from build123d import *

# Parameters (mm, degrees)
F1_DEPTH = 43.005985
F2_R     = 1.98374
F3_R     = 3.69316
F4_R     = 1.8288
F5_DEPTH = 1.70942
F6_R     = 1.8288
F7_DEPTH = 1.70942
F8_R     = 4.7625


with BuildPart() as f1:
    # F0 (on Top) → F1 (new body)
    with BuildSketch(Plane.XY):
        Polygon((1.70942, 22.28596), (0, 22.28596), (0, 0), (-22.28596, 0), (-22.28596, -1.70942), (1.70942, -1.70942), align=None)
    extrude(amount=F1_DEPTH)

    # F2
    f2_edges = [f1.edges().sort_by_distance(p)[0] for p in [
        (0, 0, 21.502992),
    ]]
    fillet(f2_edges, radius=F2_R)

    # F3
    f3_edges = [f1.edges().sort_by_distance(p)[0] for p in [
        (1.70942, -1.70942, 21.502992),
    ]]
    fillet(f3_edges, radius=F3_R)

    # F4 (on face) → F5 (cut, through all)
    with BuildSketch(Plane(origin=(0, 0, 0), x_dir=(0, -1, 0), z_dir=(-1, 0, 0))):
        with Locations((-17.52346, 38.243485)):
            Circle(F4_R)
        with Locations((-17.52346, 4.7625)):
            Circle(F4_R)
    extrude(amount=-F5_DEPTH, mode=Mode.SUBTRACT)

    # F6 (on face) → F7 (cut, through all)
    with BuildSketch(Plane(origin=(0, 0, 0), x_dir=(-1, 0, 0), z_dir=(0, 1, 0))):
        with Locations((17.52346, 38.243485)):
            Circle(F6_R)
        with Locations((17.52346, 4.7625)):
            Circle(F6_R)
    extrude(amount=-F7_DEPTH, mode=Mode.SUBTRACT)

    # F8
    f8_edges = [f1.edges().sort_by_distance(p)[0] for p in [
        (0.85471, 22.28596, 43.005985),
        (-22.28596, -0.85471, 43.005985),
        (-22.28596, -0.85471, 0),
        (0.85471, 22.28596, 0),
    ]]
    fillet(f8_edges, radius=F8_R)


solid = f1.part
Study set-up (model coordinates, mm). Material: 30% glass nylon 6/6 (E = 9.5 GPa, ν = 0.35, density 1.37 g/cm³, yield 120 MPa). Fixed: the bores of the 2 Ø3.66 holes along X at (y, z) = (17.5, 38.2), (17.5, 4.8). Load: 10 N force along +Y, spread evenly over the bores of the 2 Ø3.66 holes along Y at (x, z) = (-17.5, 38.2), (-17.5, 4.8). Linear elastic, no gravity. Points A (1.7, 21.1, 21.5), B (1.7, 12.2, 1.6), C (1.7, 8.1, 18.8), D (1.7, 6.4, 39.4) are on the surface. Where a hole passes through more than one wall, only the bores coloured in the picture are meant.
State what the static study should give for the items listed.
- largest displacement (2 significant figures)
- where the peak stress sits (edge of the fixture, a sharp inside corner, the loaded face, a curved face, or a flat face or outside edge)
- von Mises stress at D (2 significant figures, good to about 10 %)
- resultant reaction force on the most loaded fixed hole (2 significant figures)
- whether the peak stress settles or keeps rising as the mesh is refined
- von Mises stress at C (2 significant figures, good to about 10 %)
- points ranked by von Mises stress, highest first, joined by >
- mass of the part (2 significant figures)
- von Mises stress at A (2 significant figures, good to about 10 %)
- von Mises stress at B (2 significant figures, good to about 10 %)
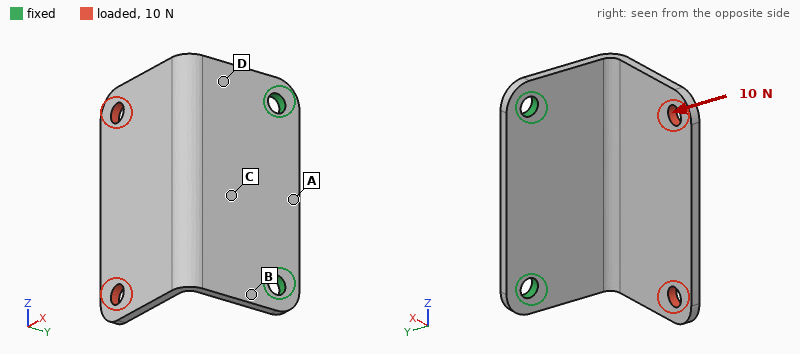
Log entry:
0.63 mm
edge of the fixture
8.7 MPa
5.4 N
keeps rising
6.6 MPa
B > D > C > A
4.4 g
2.8 MPa
11 MPa
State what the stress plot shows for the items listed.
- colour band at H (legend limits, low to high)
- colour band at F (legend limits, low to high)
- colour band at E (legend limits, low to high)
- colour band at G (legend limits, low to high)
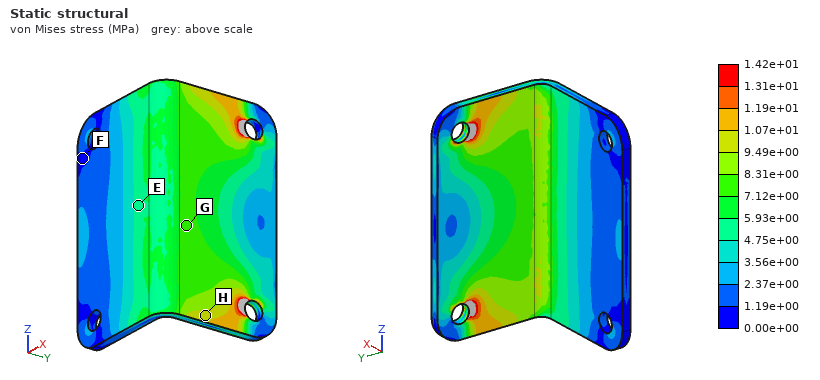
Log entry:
9.49e+00 to 1.07e+01 MPa
0.00e+00 to 1.19e+00 MPa
4.75e+00 to 5.93e+00 MPa
7.12e+00 to 8.31e+00 MPa
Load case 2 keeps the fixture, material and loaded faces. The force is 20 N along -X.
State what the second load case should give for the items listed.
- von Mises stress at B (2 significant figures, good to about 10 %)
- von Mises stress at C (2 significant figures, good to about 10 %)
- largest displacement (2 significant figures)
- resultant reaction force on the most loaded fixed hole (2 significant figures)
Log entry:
18 MPa
5.9 MPa
0.56 mm
10 N
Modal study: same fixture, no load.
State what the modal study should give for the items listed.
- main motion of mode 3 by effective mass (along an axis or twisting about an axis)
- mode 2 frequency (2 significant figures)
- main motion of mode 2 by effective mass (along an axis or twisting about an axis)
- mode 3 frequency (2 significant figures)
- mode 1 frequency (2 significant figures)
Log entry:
along X
1100 Hz
along Z
1600 Hz
580 Hz
